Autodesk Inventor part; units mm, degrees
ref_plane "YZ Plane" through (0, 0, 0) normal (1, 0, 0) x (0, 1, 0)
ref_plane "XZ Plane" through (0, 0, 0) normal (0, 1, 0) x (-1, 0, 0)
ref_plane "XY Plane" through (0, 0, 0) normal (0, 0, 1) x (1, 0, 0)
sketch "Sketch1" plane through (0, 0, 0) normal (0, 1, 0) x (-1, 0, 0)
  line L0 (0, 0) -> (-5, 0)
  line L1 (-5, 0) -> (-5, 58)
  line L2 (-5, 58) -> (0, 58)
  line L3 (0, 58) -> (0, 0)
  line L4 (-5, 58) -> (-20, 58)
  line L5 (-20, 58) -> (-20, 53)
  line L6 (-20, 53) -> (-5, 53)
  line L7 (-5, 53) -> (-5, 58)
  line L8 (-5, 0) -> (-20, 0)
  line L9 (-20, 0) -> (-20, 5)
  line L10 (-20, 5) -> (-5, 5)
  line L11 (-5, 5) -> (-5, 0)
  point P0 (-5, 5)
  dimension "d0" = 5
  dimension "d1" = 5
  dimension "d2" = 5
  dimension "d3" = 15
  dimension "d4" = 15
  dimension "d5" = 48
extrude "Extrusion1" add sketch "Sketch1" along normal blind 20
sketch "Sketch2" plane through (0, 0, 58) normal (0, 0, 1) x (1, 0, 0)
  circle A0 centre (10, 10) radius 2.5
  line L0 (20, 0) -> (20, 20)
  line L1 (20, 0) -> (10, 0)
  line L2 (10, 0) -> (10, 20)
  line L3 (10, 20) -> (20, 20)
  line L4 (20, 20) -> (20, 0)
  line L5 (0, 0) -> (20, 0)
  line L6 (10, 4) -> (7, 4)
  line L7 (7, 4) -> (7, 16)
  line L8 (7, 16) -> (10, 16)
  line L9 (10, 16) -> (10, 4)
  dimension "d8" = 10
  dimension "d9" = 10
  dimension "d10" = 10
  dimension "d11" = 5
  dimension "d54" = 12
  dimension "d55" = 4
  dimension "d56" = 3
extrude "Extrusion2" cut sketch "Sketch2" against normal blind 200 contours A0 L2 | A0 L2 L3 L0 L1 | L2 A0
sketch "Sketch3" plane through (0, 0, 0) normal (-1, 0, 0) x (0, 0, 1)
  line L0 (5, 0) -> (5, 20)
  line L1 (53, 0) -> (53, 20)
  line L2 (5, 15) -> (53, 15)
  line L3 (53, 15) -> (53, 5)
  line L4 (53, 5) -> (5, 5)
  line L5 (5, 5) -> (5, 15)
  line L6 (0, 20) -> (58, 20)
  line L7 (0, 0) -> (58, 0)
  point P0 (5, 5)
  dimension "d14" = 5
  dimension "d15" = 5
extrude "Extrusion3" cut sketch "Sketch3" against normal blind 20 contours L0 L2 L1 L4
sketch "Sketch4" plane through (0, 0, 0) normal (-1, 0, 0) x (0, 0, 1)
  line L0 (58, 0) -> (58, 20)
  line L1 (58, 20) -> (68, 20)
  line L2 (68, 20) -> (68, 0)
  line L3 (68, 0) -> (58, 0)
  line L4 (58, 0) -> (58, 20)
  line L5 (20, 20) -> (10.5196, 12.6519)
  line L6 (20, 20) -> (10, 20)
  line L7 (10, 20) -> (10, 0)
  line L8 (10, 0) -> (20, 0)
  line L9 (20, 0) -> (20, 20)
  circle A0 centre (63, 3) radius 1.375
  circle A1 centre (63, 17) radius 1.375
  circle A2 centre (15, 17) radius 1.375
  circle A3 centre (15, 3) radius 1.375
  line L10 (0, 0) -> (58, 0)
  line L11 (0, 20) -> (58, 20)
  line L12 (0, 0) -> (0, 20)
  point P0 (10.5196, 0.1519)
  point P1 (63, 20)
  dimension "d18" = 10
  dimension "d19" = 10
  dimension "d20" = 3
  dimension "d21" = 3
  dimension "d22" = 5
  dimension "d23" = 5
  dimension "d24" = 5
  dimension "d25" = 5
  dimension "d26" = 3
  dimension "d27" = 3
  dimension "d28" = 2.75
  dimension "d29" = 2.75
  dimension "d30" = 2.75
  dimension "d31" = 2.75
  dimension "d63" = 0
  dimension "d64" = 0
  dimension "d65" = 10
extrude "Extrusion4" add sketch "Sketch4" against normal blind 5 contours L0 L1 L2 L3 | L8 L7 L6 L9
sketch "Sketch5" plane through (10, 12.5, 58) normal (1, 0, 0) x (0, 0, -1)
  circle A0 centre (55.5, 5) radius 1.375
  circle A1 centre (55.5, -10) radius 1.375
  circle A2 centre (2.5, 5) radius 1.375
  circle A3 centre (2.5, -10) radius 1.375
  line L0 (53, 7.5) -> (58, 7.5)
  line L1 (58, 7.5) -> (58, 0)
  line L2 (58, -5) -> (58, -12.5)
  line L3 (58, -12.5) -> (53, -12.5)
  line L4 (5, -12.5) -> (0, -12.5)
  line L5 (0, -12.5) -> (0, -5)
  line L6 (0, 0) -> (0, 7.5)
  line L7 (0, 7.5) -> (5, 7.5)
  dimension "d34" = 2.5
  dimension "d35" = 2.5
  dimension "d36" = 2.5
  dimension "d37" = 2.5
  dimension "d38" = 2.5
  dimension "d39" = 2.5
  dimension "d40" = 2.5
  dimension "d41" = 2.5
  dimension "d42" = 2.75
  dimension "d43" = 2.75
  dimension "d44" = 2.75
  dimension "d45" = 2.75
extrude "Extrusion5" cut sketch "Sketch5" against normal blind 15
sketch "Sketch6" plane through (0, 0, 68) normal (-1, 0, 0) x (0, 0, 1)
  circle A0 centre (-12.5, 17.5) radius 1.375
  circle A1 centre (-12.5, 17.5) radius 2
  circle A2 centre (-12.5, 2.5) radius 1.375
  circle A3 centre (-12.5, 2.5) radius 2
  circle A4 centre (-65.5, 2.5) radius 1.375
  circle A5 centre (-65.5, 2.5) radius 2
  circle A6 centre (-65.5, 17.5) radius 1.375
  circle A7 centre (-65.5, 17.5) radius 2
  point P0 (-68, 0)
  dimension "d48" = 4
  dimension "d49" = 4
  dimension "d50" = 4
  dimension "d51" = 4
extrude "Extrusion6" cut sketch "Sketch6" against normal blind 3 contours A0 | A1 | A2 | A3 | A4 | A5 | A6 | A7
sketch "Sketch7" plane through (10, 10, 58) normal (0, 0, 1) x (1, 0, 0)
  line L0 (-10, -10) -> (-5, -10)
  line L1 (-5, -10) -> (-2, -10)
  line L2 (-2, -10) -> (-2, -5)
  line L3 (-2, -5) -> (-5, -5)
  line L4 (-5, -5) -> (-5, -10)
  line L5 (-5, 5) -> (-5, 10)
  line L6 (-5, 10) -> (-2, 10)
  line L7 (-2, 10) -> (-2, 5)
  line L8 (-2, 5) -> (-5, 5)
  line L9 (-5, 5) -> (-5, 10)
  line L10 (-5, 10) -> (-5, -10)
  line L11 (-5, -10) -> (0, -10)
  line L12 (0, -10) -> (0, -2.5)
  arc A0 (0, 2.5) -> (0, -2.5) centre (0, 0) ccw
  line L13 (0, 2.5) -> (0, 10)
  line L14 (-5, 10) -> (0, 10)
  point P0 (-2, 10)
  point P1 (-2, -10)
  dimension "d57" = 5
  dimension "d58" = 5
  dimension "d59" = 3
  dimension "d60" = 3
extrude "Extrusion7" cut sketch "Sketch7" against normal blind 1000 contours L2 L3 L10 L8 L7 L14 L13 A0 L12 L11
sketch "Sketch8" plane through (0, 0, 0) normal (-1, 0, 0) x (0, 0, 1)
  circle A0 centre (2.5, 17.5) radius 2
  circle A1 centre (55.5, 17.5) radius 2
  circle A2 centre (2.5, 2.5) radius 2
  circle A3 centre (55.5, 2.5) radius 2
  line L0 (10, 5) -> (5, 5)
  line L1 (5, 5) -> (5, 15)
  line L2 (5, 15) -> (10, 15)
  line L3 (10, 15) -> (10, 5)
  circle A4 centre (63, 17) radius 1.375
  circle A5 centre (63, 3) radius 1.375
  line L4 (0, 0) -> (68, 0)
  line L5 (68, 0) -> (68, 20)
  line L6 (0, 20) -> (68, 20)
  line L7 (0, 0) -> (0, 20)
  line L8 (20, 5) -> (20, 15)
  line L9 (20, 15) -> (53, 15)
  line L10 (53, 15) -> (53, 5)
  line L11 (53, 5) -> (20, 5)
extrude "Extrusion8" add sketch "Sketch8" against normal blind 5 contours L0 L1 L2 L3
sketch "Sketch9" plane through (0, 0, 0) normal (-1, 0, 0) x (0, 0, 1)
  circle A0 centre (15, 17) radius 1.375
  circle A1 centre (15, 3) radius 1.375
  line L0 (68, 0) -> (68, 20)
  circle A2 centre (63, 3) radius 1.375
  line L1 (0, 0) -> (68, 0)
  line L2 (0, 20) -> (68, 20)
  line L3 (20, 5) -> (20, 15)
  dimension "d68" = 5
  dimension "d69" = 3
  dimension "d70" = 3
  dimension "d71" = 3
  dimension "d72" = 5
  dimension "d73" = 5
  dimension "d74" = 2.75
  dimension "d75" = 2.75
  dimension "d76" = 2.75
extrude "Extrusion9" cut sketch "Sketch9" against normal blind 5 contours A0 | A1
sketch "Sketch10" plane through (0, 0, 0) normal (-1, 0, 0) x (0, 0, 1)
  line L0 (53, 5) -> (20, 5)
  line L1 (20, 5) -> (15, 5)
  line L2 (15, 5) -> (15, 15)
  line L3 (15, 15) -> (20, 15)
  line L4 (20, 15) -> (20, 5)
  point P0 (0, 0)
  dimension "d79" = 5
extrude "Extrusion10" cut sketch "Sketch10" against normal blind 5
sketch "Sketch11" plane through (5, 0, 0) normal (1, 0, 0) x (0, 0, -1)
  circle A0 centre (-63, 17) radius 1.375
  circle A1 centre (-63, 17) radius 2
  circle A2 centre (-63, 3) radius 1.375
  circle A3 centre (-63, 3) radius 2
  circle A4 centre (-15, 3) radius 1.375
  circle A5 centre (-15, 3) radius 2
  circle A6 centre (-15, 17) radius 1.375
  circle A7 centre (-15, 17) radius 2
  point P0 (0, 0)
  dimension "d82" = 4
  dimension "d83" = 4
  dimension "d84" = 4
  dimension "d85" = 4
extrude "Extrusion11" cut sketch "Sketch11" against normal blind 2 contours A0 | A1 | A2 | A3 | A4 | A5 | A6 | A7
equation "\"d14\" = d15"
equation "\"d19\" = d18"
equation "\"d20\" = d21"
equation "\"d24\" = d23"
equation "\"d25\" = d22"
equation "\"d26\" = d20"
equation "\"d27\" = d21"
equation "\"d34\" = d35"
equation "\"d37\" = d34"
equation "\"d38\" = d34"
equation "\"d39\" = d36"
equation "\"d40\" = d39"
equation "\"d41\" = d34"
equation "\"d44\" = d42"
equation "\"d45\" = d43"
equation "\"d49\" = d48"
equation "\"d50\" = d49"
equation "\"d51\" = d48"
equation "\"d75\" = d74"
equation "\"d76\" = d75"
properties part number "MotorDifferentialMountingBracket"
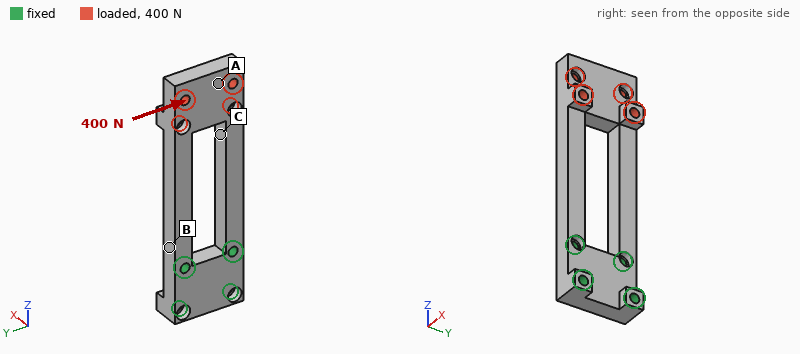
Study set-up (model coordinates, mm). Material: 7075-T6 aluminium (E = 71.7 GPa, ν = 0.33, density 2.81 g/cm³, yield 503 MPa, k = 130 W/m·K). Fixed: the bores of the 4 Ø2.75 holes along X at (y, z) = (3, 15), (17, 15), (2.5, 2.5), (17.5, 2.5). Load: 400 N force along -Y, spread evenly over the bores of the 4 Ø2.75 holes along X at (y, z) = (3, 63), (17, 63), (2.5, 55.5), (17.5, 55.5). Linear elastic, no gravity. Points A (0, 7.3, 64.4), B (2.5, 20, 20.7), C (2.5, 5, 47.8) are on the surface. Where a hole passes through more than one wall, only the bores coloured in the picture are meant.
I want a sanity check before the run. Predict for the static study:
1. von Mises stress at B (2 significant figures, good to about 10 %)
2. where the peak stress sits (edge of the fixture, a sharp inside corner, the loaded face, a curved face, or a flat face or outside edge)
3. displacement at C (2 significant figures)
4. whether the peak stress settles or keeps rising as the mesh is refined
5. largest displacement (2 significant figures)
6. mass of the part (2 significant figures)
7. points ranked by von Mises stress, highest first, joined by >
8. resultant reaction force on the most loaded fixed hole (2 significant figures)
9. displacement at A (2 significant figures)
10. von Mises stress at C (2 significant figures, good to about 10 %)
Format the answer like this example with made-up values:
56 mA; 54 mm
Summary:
180 MPa; a sharp inside corner; 0.35 mm; keeps rising; 0.43 mm; 13 g; B > C > A; 580 N; 0.40 mm; 140 MPa
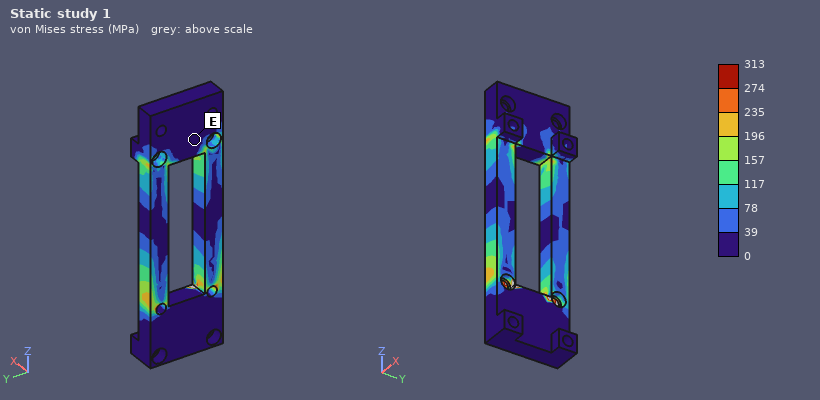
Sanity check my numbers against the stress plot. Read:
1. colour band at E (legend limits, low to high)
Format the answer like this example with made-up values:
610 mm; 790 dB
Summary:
0 to 39 MPa
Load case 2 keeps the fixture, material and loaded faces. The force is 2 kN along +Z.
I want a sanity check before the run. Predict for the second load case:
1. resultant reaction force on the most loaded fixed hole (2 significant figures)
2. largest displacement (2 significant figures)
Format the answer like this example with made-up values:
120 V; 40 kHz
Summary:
910 N; 0.65 mm
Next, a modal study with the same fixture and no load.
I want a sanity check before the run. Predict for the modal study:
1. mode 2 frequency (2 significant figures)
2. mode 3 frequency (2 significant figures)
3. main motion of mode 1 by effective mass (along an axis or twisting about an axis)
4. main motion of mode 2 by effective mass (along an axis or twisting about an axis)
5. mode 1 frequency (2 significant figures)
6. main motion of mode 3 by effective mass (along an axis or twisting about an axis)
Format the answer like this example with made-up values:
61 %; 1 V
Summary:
2100 Hz; 4000 Hz; along X; along Y; 1000 Hz; twisting about Z
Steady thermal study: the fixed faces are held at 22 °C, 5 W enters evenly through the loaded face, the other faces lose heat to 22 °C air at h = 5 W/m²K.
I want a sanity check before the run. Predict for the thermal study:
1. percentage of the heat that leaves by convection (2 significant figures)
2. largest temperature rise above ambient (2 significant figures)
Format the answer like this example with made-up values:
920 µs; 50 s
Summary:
5.5 %; 32 K
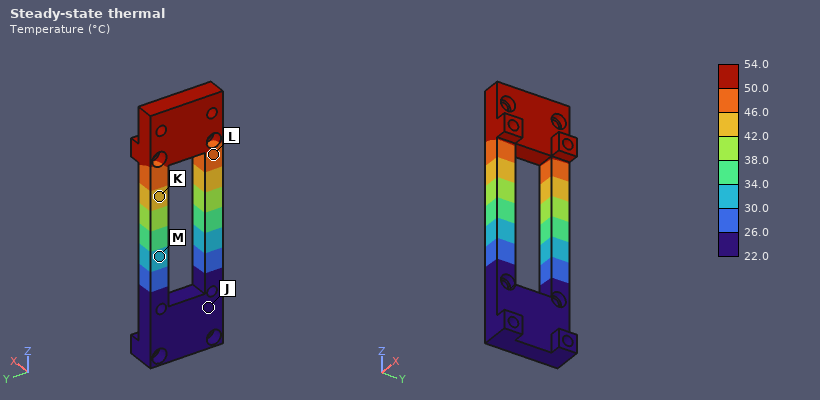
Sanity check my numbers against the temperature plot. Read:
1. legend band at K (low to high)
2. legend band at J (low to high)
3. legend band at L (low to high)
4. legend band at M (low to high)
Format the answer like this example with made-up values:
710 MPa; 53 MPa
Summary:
42.0 to 46.0 °C; 22.0 to 26.0 °C; 46.0 to 50.0 °C; 30.0 to 34.0 °C
